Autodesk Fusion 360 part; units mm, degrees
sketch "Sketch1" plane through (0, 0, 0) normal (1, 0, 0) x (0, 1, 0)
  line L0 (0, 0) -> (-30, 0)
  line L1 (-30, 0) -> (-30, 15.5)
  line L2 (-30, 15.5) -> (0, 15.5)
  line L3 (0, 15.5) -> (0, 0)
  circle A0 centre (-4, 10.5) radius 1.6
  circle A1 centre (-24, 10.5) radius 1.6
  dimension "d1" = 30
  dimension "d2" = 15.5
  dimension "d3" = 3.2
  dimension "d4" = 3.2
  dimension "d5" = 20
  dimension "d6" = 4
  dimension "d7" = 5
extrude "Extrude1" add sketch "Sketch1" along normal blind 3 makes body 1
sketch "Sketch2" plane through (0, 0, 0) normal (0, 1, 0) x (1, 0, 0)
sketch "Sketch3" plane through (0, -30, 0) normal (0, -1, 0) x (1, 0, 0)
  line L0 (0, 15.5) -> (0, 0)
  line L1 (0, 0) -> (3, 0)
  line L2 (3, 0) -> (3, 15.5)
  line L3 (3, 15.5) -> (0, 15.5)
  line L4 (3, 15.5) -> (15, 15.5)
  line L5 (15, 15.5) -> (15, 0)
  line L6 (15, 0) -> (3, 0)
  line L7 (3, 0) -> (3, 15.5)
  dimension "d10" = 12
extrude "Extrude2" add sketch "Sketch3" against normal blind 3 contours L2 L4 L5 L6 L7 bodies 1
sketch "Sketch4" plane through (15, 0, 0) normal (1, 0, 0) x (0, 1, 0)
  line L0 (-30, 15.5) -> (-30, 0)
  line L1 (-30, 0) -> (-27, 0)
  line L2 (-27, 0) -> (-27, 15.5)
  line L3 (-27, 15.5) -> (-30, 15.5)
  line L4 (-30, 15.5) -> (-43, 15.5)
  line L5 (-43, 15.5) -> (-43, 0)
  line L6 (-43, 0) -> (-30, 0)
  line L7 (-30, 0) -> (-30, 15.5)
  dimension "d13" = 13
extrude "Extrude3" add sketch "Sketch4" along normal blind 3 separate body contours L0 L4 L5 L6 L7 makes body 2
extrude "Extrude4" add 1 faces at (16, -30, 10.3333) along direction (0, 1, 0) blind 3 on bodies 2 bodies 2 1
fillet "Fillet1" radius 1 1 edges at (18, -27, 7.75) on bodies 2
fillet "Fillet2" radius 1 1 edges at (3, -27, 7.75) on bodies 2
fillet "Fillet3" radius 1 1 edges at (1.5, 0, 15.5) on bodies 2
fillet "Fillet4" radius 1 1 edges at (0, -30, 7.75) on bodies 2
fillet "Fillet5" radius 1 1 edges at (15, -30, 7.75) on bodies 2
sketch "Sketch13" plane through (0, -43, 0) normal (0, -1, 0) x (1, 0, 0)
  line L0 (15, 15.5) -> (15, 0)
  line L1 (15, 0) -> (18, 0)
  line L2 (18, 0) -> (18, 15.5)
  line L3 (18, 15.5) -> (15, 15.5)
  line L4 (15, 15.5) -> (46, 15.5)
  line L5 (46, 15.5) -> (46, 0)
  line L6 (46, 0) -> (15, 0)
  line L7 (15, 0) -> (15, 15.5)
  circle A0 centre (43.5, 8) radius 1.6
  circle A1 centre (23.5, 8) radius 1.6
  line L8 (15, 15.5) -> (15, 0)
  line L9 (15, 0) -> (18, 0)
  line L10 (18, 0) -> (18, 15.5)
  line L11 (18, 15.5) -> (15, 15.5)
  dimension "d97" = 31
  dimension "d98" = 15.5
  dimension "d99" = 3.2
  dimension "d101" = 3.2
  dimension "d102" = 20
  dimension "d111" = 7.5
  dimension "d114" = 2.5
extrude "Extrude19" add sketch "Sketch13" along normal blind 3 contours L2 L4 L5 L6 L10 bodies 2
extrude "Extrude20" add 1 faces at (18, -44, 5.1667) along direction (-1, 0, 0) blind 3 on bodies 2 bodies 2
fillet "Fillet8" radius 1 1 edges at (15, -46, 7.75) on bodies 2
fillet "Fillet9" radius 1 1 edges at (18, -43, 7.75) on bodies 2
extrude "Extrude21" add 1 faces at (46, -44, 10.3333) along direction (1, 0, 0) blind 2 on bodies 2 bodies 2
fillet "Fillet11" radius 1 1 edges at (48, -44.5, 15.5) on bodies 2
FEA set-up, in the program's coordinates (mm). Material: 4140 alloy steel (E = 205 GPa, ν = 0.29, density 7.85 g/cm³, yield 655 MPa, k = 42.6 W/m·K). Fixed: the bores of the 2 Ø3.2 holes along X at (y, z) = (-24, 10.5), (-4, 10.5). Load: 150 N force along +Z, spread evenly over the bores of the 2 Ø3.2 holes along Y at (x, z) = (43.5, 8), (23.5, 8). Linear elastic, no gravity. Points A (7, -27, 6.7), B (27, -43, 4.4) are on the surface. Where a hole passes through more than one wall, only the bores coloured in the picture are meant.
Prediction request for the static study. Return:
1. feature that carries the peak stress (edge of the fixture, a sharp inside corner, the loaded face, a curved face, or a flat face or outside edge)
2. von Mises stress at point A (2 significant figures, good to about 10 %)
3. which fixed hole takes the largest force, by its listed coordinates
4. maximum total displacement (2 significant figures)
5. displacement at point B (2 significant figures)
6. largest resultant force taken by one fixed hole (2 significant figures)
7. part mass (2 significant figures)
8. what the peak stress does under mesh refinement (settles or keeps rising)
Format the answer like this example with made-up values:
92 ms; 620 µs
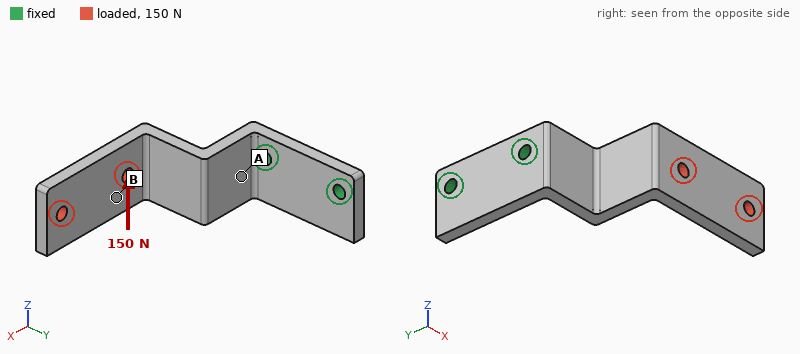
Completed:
edge of the fixture; 53 MPa; (-24, 10.5); 0.18 mm; 0.092 mm; 270 N; 32 g; keeps rising
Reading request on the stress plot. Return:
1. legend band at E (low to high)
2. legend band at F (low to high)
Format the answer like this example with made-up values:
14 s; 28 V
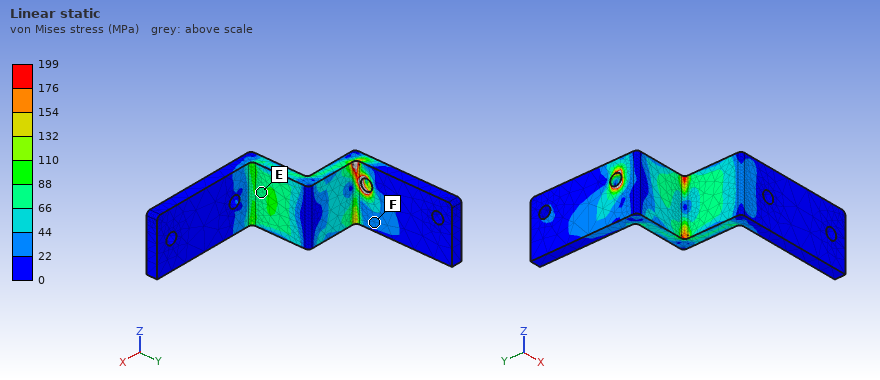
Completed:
66 to 88 MPa; 22 to 44 MPa
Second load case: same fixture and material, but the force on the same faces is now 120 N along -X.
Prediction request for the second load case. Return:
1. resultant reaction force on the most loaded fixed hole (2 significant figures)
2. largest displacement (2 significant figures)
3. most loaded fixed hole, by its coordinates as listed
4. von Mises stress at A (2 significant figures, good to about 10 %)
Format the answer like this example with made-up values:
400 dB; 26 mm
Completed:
150 N; 0.27 mm; (-24, 10.5); 71 MPa
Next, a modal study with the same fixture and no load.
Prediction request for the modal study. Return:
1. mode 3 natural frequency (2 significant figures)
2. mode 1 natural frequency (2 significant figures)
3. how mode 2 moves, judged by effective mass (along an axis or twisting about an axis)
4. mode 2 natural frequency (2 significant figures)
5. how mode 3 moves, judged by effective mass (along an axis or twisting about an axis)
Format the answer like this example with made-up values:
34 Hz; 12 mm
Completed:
3500 Hz; 800 Hz; along Z; 1600 Hz; along X
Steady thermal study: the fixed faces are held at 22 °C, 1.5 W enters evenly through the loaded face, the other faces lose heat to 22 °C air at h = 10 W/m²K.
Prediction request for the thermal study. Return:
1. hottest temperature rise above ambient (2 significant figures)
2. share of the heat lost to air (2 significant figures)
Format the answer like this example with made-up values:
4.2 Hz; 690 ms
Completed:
30 K; 28 %
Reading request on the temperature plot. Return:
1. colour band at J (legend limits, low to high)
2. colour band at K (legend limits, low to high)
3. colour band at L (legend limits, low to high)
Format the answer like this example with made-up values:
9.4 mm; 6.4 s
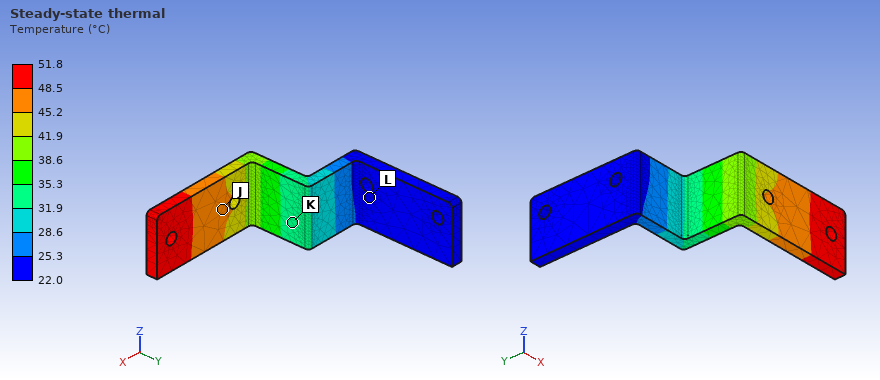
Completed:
45.2 to 48.5 °C; 31.9 to 35.3 °C; 22.0 to 25.3 °C
